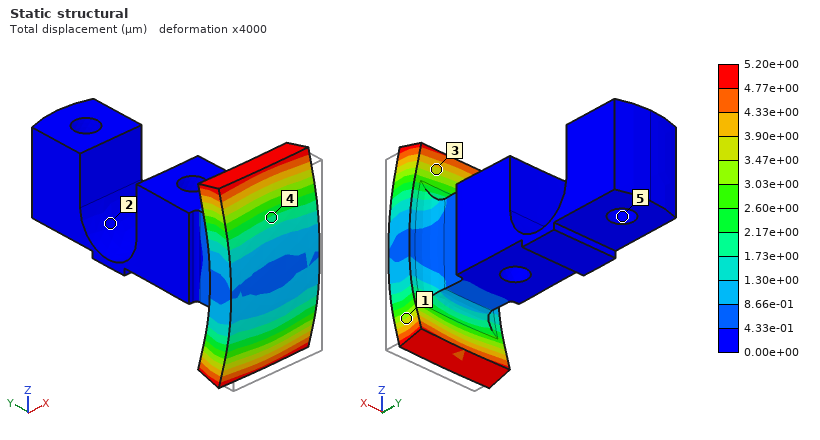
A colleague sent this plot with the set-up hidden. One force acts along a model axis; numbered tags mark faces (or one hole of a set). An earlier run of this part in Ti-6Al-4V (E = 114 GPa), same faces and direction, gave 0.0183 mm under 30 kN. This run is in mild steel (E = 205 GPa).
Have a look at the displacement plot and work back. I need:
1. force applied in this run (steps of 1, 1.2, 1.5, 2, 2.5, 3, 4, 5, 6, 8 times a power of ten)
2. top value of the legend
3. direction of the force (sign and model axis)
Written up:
15 kN
5.20e+00 µm
+Y
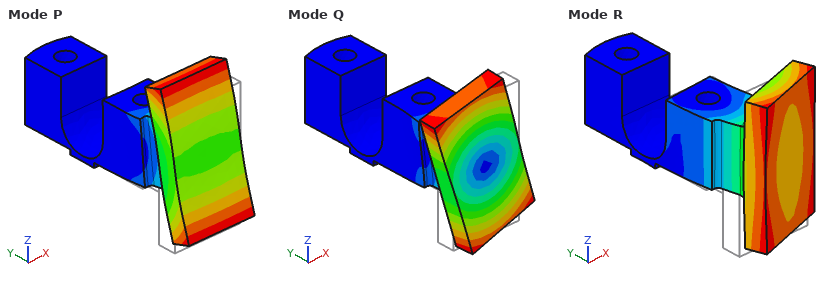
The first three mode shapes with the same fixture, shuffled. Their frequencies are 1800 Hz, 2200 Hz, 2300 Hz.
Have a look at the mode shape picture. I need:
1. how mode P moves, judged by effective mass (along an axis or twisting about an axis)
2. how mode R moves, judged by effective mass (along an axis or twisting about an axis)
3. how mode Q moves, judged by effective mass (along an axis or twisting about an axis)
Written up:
along Z
along X
twisting about Y
